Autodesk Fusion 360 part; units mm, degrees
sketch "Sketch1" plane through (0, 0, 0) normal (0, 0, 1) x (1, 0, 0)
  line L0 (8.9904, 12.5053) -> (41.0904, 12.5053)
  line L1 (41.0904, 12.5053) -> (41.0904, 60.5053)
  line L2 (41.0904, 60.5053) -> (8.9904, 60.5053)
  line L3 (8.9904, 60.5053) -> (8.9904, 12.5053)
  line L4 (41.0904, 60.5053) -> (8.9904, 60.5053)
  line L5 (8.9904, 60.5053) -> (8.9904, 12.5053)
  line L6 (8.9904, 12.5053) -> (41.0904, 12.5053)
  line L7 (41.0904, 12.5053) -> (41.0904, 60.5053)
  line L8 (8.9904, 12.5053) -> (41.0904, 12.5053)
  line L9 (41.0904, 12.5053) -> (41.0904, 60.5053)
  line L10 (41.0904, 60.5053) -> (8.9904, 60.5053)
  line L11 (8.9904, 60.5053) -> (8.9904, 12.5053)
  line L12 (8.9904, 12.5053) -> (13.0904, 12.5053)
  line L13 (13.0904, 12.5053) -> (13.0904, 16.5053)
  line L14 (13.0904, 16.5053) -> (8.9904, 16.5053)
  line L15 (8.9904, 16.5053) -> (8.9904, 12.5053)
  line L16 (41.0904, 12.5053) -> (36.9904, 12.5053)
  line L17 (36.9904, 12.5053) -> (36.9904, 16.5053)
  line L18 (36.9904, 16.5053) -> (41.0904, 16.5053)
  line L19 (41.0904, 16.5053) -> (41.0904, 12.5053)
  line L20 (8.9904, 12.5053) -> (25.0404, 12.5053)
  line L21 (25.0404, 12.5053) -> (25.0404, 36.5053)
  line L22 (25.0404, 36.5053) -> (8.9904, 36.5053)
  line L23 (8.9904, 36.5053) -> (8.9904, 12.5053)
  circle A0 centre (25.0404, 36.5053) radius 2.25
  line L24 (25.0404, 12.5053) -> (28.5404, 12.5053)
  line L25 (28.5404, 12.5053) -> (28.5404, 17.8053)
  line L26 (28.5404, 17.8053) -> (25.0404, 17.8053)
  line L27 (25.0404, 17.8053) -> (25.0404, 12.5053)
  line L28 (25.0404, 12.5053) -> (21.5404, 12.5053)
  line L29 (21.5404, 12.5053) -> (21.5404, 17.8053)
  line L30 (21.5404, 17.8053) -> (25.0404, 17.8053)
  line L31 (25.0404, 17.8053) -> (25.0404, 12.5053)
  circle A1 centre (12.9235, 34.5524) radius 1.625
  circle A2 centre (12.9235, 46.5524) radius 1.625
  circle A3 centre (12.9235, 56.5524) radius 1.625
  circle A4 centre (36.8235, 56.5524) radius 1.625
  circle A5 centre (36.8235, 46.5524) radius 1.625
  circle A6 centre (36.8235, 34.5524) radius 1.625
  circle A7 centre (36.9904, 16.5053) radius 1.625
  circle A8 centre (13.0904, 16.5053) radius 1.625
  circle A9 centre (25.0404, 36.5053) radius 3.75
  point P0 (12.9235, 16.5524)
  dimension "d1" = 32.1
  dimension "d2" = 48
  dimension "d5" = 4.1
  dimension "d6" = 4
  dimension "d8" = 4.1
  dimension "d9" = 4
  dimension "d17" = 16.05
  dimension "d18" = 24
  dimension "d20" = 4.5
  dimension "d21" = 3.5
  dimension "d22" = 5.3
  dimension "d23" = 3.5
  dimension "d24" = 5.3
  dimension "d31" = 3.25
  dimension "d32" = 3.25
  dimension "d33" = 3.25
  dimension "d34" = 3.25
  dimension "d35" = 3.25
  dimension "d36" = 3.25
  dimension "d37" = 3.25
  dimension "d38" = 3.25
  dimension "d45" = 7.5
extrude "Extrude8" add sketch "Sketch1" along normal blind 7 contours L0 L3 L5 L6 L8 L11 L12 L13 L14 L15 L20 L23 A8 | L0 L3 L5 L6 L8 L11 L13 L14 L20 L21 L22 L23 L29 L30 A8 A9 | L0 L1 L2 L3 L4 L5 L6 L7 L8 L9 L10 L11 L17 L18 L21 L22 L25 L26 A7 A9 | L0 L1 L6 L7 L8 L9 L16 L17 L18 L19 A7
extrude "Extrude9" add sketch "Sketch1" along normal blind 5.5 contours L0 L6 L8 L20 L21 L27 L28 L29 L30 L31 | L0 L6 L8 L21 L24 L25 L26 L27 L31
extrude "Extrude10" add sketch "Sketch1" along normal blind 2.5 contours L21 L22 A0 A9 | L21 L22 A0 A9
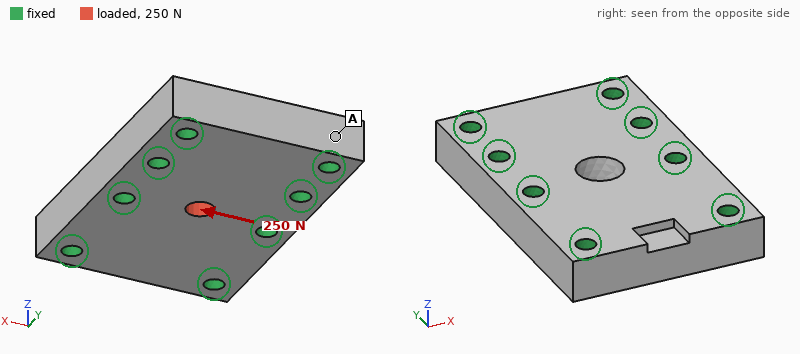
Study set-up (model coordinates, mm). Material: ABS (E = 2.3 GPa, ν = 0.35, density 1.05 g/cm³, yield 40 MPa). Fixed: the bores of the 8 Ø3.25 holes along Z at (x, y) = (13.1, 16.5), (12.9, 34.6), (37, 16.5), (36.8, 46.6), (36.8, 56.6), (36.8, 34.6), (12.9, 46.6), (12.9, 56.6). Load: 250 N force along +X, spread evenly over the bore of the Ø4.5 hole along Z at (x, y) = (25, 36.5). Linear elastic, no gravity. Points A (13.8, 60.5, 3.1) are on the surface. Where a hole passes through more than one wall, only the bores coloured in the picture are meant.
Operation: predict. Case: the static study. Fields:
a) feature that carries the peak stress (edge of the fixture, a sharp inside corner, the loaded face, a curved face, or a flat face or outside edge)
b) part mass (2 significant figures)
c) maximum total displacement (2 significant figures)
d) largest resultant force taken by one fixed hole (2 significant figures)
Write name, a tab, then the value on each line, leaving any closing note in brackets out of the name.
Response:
feature that carries the peak stress	the loaded face
part mass	11 g
maximum total displacement	18 µm
largest resultant force taken by one fixed hole	81 N
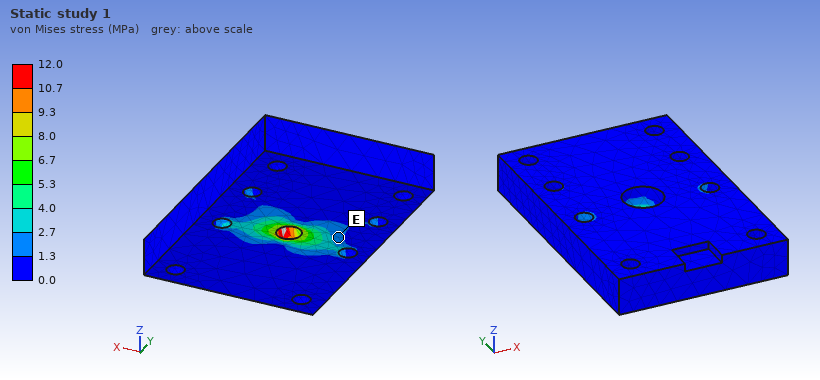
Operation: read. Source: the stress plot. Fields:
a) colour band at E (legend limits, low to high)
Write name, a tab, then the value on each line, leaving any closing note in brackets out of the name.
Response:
colour band at E	1.3 to 2.7 MPa
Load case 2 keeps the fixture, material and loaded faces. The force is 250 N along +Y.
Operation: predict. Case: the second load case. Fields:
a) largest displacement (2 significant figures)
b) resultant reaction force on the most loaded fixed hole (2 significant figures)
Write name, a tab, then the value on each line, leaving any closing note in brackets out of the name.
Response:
largest displacement	20 µm
resultant reaction force on the most loaded fixed hole	45 N
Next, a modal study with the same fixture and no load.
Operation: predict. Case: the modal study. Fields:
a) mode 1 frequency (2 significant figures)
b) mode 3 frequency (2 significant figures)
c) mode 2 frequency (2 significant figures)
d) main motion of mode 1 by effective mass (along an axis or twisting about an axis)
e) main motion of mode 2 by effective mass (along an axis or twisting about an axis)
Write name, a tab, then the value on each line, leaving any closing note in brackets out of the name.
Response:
mode 1 frequency	12 kHz
mode 3 frequency	16 kHz
mode 2 frequency	14 kHz
main motion of mode 1 by effective mass	along Z
main motion of mode 2 by effective mass	along Z
